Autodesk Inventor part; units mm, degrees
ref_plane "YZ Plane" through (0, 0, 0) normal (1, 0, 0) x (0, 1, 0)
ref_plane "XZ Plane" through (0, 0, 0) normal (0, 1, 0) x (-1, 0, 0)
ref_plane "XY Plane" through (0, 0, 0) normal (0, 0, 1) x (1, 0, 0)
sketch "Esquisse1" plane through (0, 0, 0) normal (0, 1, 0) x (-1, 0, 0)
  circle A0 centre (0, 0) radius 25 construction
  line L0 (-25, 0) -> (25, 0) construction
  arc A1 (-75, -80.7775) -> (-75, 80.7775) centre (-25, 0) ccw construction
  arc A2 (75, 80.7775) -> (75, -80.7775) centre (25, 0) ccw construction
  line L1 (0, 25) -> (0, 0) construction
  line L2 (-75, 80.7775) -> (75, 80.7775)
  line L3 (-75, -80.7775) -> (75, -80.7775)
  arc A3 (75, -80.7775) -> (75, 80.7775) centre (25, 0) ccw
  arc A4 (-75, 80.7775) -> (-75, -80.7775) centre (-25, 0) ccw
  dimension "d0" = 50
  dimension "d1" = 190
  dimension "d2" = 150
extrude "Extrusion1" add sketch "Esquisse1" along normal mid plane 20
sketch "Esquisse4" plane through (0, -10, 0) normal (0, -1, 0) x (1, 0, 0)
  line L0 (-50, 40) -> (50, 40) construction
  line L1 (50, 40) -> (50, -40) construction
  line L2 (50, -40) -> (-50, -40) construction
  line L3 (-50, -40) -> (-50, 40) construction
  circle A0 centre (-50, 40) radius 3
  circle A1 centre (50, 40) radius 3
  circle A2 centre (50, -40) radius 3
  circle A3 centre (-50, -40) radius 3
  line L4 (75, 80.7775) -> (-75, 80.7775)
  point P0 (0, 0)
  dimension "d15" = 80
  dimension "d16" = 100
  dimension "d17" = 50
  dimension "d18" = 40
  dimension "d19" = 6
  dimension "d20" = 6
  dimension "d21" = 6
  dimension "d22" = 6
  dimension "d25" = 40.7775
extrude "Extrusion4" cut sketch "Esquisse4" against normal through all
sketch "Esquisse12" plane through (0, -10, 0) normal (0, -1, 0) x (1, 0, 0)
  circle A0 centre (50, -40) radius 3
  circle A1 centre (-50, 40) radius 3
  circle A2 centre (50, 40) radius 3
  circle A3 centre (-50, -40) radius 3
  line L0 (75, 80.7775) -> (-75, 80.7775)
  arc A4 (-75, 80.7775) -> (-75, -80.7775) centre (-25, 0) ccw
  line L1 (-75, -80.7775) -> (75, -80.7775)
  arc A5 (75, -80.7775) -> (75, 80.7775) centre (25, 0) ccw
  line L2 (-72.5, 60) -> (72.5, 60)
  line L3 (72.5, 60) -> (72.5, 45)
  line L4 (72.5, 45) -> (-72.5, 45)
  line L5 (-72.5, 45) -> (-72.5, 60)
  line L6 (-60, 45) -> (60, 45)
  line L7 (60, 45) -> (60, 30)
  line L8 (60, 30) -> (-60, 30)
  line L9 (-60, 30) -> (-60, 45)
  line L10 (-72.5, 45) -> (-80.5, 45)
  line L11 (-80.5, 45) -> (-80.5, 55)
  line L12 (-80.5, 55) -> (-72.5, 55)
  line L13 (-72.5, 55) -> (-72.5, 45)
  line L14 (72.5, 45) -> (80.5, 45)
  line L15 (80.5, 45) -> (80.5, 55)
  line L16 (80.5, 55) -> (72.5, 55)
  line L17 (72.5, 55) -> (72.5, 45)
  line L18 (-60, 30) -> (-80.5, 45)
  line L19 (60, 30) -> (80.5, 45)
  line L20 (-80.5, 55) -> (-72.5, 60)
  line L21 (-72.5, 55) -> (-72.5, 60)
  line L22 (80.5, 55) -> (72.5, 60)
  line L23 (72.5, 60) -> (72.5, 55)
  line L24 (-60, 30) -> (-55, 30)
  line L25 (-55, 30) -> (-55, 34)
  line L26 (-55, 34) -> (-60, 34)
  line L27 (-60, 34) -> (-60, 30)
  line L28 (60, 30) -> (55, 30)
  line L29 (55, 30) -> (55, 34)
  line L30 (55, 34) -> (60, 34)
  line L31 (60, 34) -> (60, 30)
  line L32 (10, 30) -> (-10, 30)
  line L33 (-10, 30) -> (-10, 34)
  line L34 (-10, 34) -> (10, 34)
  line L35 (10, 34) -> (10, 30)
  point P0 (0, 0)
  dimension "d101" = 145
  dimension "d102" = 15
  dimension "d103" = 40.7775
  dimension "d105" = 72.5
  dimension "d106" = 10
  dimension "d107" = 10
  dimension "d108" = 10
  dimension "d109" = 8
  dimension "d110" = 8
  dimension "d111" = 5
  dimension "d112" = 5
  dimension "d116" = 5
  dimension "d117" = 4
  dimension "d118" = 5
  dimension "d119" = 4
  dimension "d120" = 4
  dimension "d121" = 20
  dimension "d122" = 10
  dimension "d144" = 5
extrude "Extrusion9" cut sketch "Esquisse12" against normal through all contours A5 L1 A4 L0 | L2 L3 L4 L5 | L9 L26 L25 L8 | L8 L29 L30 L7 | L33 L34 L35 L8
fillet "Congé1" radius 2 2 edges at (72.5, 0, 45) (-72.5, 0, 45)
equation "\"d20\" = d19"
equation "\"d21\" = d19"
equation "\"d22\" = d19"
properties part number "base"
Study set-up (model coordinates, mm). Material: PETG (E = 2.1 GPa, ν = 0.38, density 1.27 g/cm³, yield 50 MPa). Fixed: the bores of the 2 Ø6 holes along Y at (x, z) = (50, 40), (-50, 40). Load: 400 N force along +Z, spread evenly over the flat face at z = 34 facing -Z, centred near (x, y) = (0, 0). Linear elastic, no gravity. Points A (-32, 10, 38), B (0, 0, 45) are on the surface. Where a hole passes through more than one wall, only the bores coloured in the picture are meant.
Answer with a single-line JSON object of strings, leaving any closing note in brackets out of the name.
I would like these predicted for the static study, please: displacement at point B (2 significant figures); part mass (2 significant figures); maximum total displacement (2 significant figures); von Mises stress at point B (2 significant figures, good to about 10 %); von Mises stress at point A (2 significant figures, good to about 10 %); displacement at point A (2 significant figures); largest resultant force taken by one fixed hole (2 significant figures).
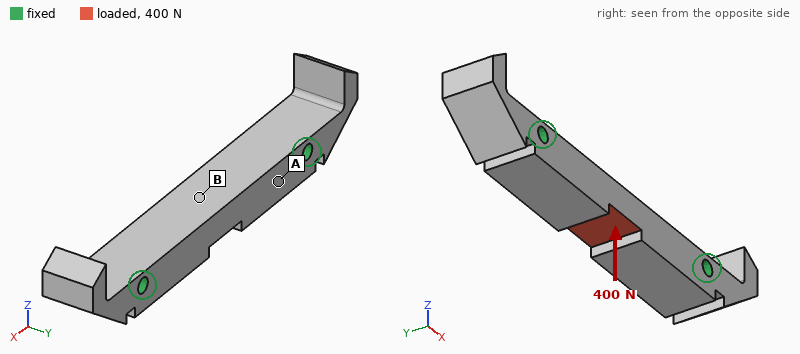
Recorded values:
{"displacement at point B": "0.35 mm", "part mass": "54 g", "maximum total displacement": "0.36 mm", "von Mises stress at point B": "8.0 MPa", "von Mises stress at point A": "2.1 MPa", "displacement at point A": "0.11 mm", "largest resultant force taken by one fixed hole": "210 N"}
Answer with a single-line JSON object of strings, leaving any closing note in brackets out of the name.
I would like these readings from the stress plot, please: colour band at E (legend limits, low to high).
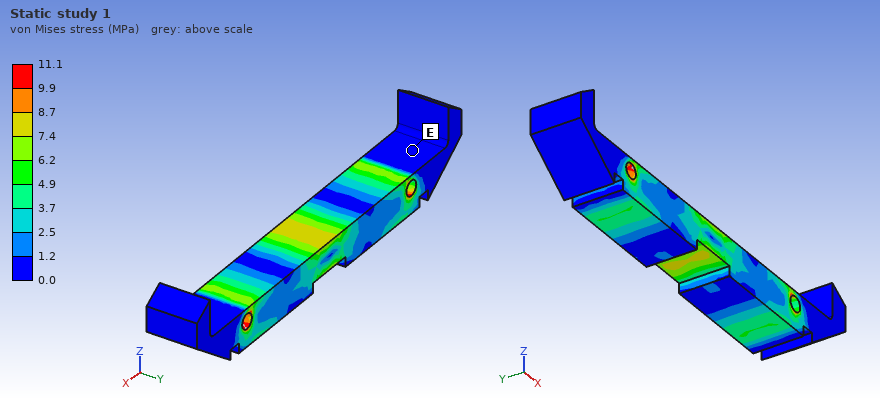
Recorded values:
{"colour band at E": "0.0 to 1.2 MPa"}
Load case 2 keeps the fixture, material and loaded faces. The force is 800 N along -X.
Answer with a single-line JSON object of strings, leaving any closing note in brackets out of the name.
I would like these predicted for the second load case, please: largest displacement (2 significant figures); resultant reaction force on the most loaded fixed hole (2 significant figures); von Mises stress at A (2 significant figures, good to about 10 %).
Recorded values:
{"largest displacement": "48 µm", "resultant reaction force on the most loaded fixed hole": "400 N", "von Mises stress at A": "1.4 MPa"}
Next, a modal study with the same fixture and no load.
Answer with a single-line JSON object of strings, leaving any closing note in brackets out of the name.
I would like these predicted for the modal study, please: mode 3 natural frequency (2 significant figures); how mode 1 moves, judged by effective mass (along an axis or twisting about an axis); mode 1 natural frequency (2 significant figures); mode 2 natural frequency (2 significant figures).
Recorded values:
{"mode 3 natural frequency": "1800 Hz", "how mode 1 moves, judged by effective mass": "along Z", "mode 1 natural frequency": "1400 Hz", "mode 2 natural frequency": "1700 Hz"}
